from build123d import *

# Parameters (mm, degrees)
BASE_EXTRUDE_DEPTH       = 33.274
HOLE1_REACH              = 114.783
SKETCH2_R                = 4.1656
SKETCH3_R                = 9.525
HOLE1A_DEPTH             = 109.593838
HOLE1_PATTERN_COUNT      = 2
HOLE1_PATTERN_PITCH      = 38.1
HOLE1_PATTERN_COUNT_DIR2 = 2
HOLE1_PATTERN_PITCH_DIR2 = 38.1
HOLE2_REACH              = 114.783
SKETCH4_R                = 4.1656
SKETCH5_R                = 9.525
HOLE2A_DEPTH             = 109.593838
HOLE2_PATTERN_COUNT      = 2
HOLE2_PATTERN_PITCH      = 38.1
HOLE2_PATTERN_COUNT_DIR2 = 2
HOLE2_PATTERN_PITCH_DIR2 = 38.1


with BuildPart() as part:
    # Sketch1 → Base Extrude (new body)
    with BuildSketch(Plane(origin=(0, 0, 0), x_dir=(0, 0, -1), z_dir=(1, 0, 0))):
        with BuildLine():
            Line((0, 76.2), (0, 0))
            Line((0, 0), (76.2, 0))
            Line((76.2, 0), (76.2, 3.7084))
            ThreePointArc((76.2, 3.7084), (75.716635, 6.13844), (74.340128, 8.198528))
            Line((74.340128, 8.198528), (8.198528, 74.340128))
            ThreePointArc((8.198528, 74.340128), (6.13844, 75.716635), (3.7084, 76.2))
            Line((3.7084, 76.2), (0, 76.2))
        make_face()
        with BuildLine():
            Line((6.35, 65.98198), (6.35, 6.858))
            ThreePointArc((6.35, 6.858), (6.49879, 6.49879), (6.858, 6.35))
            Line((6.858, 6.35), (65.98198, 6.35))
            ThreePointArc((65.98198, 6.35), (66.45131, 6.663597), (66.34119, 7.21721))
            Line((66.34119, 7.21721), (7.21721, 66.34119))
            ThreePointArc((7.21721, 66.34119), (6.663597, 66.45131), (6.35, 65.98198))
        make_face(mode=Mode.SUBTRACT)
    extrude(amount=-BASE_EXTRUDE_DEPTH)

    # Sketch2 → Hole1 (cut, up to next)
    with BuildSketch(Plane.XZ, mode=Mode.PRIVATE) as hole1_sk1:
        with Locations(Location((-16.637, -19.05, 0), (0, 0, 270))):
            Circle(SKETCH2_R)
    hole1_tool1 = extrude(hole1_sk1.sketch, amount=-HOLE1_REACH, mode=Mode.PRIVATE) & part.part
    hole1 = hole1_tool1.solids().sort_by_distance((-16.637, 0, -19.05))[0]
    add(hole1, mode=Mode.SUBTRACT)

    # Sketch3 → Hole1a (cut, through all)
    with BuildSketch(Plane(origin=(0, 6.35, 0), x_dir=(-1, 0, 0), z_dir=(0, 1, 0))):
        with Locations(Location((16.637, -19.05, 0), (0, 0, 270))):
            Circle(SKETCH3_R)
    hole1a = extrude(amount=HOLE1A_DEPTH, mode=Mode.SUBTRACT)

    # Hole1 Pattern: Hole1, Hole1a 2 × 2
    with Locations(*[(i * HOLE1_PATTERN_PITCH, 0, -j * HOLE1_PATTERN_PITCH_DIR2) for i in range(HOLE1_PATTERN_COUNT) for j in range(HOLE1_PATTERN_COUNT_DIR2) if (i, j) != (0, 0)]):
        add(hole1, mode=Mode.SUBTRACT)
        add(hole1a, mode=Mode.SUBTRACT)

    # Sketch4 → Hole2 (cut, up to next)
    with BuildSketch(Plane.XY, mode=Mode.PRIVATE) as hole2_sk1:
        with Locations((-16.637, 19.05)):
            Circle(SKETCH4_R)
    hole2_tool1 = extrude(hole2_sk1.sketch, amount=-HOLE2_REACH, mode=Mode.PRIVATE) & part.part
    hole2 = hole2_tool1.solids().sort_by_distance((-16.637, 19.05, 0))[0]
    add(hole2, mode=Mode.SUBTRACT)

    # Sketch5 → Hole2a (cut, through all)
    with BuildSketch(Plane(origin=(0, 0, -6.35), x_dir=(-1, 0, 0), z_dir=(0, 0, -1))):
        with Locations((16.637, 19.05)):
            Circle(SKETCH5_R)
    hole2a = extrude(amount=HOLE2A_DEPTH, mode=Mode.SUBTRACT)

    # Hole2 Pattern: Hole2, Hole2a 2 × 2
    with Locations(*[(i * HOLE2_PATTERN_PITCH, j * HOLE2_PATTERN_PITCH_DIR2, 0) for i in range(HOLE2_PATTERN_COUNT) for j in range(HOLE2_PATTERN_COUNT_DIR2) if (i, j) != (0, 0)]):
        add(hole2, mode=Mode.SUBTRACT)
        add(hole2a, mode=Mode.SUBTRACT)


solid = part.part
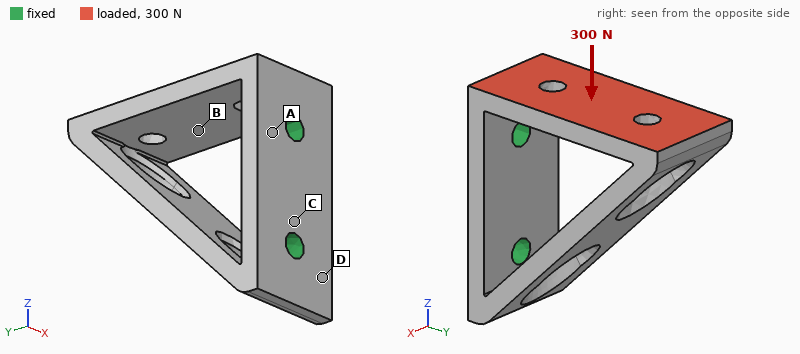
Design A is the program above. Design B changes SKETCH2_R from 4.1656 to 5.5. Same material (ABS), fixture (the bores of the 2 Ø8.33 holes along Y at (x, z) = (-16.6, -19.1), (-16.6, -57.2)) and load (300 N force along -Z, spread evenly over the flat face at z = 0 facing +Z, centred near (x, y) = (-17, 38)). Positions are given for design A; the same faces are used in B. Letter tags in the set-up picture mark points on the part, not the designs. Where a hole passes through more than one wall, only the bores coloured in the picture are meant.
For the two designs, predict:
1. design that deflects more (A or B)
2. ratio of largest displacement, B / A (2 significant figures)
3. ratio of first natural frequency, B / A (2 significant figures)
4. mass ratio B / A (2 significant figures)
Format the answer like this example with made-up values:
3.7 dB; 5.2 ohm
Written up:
A; 0.91; 1.1; 0.99
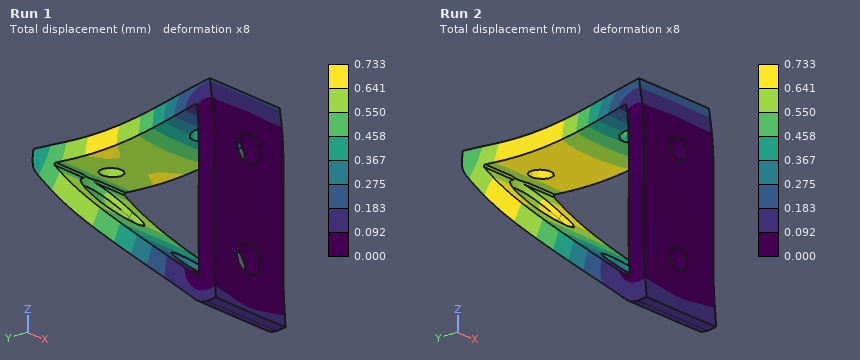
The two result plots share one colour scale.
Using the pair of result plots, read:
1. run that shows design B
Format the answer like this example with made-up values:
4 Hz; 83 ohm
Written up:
Run 1
